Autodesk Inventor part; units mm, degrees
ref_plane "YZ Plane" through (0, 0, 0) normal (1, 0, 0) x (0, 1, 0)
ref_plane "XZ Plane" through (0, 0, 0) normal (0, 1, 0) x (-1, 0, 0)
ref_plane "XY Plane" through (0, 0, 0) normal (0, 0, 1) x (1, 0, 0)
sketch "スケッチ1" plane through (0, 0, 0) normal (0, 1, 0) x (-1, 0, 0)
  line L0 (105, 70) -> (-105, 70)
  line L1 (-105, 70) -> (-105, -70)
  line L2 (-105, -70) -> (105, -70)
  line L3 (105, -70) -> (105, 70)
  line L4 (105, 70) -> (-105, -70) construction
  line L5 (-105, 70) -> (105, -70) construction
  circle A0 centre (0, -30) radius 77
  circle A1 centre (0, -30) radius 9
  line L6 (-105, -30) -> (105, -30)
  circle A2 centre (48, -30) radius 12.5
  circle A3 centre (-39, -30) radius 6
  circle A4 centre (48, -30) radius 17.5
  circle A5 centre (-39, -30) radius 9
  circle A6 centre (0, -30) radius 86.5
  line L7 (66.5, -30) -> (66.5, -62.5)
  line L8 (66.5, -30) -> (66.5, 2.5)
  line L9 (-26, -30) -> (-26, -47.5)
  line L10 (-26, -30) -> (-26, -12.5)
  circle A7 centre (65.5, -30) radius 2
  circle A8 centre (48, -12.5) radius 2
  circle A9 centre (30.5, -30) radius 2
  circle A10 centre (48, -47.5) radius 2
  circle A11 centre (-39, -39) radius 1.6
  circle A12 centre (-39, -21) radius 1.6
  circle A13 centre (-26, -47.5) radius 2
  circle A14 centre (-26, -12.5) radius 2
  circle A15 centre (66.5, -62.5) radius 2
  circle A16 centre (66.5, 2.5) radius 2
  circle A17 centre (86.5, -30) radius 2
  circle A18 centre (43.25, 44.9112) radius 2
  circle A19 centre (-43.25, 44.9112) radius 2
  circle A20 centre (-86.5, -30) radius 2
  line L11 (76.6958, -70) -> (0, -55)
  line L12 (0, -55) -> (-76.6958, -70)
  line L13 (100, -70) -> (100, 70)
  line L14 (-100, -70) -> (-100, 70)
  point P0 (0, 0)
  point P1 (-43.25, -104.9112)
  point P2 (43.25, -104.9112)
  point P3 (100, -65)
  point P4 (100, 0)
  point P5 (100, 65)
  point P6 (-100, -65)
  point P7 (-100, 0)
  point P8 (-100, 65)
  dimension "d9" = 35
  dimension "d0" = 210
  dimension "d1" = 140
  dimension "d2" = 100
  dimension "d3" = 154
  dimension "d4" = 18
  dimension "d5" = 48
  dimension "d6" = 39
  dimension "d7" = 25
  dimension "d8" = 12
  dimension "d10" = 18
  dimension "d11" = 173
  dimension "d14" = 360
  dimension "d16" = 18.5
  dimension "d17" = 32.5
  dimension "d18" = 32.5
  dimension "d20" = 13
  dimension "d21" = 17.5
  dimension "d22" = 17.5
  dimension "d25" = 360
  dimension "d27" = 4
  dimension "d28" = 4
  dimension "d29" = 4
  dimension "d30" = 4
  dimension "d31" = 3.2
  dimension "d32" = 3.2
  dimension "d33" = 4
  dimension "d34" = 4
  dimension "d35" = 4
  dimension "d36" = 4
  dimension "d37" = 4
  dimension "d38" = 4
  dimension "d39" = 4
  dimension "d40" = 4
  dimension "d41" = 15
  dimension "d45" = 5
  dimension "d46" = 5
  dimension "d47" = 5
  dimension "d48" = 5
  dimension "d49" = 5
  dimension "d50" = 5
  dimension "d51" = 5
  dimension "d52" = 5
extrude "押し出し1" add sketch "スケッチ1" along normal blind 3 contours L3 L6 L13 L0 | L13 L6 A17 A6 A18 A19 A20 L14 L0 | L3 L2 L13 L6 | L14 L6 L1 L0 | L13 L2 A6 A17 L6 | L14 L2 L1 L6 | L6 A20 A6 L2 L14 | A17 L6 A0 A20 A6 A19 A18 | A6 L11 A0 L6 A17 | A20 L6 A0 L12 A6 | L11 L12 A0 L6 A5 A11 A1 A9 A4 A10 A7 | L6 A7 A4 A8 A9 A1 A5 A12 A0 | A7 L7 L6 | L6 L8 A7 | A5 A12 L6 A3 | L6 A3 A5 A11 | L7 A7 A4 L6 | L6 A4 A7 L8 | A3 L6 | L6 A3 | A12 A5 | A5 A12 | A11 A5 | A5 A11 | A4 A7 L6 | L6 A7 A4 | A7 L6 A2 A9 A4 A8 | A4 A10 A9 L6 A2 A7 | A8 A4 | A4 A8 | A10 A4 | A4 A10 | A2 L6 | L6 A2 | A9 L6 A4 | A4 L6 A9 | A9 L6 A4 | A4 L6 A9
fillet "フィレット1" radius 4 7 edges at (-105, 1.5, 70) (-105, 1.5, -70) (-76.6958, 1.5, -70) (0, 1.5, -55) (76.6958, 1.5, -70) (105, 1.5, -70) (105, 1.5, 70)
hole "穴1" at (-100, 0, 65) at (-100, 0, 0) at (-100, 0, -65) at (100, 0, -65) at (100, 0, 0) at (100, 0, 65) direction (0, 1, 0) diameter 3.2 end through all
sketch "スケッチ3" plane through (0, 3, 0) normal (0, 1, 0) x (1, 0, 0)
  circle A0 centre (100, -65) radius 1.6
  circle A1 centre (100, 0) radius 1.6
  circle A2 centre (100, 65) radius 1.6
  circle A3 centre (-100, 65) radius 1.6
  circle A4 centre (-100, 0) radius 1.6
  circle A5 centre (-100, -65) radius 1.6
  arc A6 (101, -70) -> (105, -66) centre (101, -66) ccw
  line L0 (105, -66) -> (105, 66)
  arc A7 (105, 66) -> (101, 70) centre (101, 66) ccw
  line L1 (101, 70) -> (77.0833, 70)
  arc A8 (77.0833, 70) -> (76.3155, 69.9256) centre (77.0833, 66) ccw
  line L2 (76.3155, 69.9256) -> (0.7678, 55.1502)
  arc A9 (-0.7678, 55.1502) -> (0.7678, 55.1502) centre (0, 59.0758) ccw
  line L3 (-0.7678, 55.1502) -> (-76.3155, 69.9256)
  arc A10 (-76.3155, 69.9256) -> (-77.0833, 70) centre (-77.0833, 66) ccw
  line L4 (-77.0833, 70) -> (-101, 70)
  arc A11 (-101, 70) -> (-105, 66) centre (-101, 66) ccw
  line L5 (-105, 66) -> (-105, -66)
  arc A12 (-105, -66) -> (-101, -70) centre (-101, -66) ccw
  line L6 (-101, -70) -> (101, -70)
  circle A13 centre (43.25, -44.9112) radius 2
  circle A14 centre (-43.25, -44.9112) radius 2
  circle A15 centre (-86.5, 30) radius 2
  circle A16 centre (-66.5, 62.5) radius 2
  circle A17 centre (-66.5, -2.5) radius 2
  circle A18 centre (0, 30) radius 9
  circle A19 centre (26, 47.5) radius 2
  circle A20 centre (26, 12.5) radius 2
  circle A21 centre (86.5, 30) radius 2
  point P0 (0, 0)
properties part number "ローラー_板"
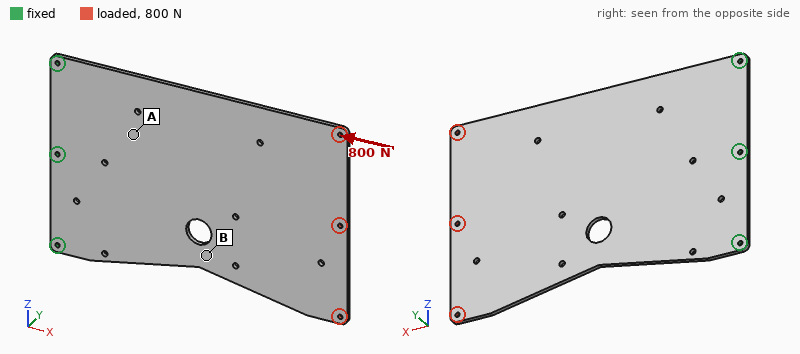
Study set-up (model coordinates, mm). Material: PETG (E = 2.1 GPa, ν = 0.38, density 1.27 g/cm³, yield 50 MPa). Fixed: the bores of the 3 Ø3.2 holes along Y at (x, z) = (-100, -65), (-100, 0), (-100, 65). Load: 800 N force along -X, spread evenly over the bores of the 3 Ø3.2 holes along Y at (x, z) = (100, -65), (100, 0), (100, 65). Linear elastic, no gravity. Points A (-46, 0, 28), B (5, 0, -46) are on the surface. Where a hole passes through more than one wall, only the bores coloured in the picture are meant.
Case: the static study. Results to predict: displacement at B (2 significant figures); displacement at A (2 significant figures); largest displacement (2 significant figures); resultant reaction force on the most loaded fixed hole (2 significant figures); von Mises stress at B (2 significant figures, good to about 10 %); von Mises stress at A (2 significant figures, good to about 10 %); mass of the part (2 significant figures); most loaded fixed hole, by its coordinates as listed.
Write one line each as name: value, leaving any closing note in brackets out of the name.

displacement at B: 0.17 mm
displacement at A: 0.094 mm
largest displacement: 0.43 mm
resultant reaction force on the most loaded fixed hole: 340 N
von Mises stress at B: 3.8 MPa
von Mises stress at A: 1.7 MPa
mass of the part: 110 g
most loaded fixed hole, by its coordinates as listed: (-100, 0)
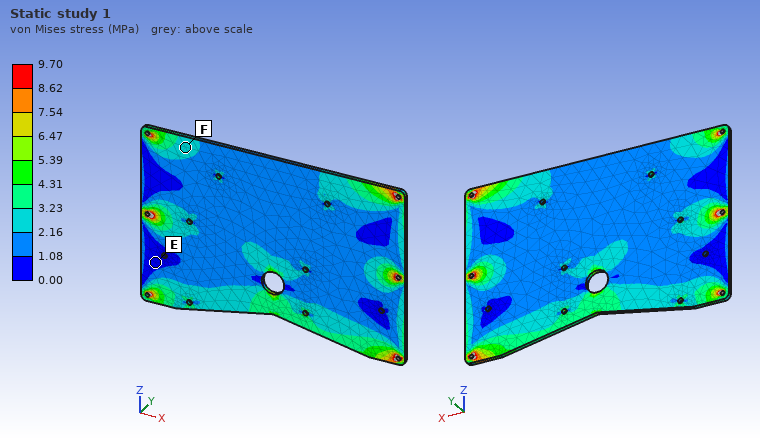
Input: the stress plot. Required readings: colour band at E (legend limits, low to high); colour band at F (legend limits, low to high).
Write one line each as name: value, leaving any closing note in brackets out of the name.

colour band at E: 0.00 to 1.08 MPa
colour band at F: 2.16 to 3.23 MPa
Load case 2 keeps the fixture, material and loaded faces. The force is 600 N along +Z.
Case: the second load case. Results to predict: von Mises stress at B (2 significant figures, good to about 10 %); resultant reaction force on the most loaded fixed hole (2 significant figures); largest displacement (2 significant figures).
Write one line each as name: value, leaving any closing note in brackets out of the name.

von Mises stress at B: 7.8 MPa
resultant reaction force on the most loaded fixed hole: 990 N
largest displacement: 2.5 mm
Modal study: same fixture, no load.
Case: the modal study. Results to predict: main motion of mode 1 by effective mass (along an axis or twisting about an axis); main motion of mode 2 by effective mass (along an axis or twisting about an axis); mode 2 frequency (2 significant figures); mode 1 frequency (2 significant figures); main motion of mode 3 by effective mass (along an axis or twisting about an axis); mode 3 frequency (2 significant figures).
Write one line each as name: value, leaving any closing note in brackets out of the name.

main motion of mode 1 by effective mass: along Y
main motion of mode 2 by effective mass: twisting about X
mode 2 frequency: 48 Hz
mode 1 frequency: 14 Hz
main motion of mode 3 by effective mass: along Y
mode 3 frequency: 87 Hz
